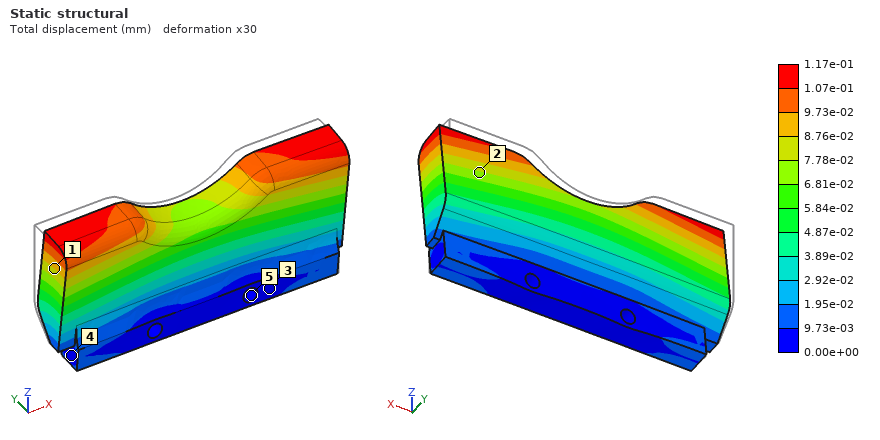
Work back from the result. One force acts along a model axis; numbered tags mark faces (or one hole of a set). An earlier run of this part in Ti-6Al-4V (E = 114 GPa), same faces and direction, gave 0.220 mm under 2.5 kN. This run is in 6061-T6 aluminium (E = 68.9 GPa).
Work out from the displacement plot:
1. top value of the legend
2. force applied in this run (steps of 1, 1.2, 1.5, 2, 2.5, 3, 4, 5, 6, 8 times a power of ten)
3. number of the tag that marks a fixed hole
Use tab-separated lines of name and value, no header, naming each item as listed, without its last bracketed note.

top value of the legend	1.17e-01 mm
force applied in this run	800 N
number of the tag that marks a fixed hole	5
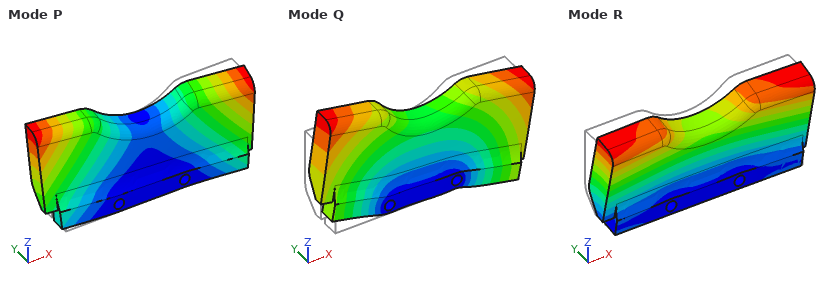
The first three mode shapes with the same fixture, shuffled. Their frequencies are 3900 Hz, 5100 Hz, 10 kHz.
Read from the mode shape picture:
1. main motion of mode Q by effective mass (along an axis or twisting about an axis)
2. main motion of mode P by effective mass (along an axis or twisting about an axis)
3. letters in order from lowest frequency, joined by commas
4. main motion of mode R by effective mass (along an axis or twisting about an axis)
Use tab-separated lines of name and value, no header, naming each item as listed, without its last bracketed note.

main motion of mode Q by effective mass	along X
main motion of mode P by effective mass	twisting about Z
letters in order from lowest frequency, joined by commas	R, P, Q
main motion of mode R by effective mass	along Y
